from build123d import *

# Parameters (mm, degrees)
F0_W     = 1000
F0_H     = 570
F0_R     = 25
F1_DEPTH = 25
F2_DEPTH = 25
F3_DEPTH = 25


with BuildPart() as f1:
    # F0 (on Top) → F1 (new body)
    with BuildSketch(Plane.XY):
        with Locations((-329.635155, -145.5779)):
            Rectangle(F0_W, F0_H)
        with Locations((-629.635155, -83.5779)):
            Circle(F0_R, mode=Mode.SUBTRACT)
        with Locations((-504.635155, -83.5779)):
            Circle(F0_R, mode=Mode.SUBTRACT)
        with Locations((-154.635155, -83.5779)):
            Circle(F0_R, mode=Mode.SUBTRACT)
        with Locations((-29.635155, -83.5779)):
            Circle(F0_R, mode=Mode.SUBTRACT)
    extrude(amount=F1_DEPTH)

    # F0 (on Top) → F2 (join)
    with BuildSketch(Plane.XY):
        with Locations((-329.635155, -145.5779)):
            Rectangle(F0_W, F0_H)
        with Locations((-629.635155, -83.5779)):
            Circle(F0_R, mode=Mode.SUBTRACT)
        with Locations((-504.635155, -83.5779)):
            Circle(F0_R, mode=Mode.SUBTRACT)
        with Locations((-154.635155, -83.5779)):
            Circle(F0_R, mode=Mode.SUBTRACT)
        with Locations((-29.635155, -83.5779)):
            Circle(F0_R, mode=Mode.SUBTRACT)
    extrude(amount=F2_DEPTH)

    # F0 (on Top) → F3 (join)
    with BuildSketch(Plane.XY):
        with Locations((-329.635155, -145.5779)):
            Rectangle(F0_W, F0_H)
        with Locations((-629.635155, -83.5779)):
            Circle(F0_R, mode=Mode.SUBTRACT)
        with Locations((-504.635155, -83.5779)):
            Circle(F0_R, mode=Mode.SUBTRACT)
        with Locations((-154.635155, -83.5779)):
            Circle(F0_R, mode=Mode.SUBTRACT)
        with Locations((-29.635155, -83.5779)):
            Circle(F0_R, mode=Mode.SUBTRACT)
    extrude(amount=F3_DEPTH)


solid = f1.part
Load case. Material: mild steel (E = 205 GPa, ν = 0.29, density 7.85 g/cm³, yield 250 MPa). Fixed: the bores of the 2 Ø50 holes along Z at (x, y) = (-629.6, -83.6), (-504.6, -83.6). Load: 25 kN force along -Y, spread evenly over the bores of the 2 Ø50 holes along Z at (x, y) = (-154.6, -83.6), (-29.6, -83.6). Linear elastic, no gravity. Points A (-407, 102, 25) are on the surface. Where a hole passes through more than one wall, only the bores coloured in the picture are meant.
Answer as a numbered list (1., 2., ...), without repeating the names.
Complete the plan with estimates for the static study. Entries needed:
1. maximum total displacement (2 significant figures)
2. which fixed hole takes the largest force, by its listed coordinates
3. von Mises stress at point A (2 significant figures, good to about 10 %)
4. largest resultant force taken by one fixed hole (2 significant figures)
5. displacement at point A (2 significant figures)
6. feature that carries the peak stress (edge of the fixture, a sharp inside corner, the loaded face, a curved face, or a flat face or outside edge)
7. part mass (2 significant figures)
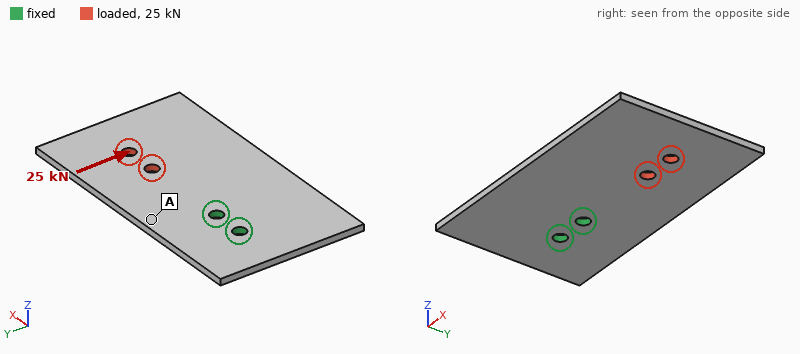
1. 0.12 mm
2. (-504.6, -83.6)
3. 6.5 MPa
4. 82 kN
5. 0.032 mm
6. edge of the fixture
7. 110 kg
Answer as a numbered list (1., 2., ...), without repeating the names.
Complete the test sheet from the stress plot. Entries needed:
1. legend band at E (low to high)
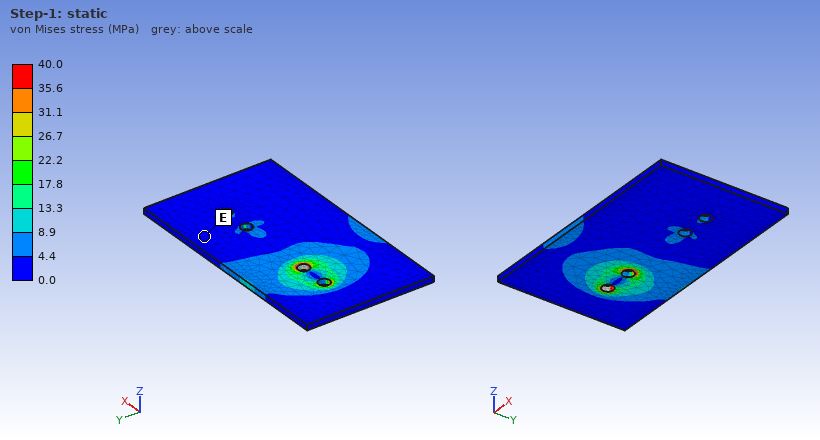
1. 0.0 to 4.4 MPa
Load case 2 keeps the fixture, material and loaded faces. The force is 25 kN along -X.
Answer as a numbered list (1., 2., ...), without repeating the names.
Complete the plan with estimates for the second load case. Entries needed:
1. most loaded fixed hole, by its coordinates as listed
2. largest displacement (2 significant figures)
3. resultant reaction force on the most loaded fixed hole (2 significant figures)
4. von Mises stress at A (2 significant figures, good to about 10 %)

1. (-504.6, -83.6)
2. 7.6 µm
3. 17 kN
4. 1.6 MPa
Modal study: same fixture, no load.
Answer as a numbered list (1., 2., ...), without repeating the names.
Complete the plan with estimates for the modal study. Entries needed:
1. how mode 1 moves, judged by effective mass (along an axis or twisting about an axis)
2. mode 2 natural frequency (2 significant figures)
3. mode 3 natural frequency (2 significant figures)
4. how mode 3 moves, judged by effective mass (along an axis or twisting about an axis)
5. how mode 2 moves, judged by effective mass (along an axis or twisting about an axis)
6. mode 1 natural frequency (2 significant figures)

1. along Z
2. 95 Hz
3. 190 Hz
4. along Z
5. twisting about X
6. 43 Hz
